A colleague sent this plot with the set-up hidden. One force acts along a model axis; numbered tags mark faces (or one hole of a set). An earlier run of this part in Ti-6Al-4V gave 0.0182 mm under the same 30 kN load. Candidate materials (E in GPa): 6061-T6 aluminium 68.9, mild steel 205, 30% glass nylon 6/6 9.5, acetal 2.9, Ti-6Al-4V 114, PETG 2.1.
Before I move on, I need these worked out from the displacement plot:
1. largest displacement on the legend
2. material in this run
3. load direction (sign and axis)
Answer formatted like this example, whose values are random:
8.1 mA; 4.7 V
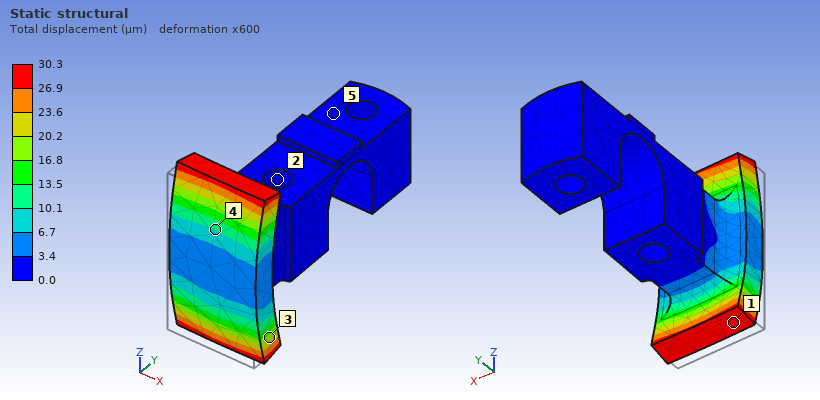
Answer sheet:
30.3 µm; 6061-T6 aluminium; +Y
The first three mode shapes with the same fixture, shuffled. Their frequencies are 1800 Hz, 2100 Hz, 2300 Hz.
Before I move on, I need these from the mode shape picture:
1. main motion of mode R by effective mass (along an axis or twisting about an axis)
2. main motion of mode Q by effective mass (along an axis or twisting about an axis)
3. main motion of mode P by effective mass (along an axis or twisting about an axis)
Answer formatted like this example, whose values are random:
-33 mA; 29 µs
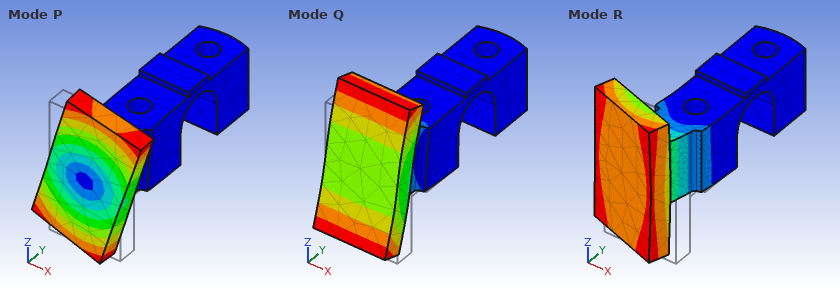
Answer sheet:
along X; along Z; twisting about Y
